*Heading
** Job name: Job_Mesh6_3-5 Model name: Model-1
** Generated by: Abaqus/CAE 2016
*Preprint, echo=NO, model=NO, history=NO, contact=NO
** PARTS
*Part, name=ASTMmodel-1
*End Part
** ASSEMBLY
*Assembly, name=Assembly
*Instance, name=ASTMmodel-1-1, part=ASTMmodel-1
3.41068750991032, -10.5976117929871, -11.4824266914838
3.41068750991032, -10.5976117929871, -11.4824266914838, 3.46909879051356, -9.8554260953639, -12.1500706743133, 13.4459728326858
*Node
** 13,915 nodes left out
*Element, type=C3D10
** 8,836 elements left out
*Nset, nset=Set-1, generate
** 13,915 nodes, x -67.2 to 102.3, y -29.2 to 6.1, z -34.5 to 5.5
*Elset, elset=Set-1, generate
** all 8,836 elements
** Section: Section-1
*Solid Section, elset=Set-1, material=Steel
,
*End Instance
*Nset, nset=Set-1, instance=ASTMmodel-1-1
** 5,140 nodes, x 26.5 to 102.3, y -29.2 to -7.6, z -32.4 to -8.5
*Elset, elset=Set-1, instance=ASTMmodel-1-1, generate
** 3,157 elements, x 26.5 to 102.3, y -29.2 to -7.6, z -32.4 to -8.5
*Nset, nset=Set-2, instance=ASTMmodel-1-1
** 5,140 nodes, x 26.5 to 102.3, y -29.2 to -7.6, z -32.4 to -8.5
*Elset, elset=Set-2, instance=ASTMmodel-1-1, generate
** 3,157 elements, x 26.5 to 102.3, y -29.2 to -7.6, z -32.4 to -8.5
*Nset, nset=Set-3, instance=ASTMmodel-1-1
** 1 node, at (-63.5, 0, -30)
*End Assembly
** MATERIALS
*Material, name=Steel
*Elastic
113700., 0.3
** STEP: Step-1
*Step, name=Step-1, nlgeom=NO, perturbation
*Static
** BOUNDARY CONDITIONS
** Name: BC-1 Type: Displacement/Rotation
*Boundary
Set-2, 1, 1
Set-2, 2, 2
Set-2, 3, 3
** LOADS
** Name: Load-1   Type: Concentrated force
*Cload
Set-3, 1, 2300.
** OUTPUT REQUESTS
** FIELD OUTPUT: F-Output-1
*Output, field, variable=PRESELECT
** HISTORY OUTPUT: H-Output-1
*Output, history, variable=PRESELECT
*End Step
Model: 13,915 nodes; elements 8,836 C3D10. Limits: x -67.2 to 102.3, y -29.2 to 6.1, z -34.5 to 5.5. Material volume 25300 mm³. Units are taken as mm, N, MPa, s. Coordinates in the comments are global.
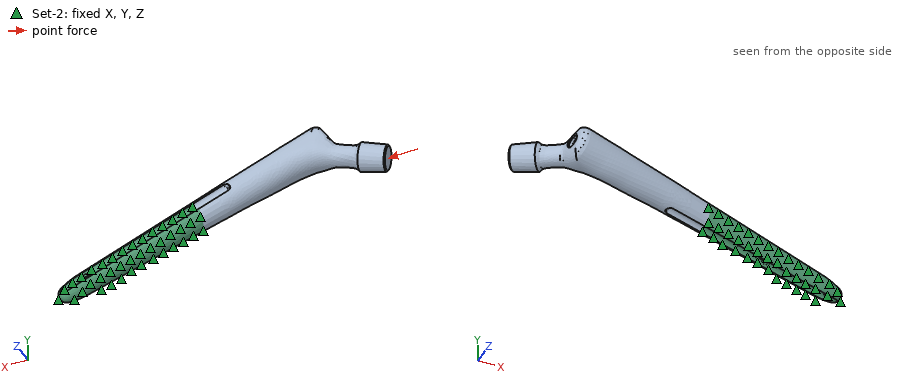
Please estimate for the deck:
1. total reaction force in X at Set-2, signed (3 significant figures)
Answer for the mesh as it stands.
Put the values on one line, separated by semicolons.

-2300 N
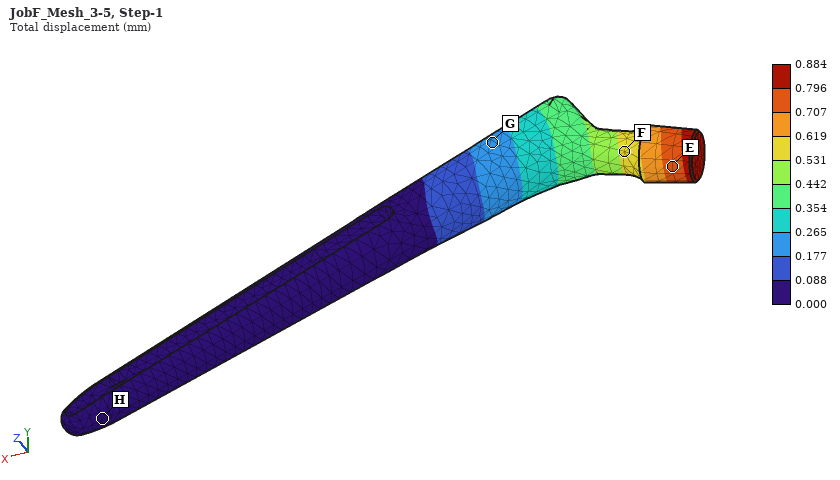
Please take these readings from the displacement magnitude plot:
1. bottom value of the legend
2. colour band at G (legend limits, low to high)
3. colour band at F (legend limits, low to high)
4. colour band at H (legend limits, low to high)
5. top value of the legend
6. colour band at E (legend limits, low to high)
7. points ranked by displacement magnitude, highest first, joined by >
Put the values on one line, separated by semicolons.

0.000 mm; 0.177 to 0.265 mm; 0.531 to 0.619 mm; 0.000 to 0.088 mm; 0.884 mm; 0.707 to 0.796 mm; E > F > G > H
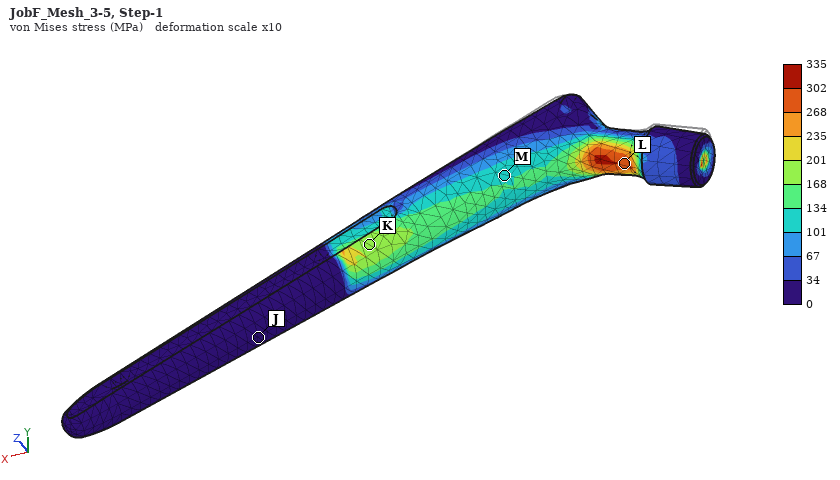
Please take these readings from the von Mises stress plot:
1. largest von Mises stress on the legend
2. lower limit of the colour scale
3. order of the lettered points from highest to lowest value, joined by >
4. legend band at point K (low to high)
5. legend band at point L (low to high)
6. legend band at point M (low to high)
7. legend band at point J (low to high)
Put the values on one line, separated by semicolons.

335 MPa; 0 MPa; L > K > M > J; 168 to 201 MPa; 268 to 302 MPa; 101 to 134 MPa; 0 to 34 MPa
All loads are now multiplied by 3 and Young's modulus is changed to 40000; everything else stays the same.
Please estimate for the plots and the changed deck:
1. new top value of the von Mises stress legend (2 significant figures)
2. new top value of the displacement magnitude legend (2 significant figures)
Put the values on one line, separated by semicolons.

1000 MPa; 7.5 mm
